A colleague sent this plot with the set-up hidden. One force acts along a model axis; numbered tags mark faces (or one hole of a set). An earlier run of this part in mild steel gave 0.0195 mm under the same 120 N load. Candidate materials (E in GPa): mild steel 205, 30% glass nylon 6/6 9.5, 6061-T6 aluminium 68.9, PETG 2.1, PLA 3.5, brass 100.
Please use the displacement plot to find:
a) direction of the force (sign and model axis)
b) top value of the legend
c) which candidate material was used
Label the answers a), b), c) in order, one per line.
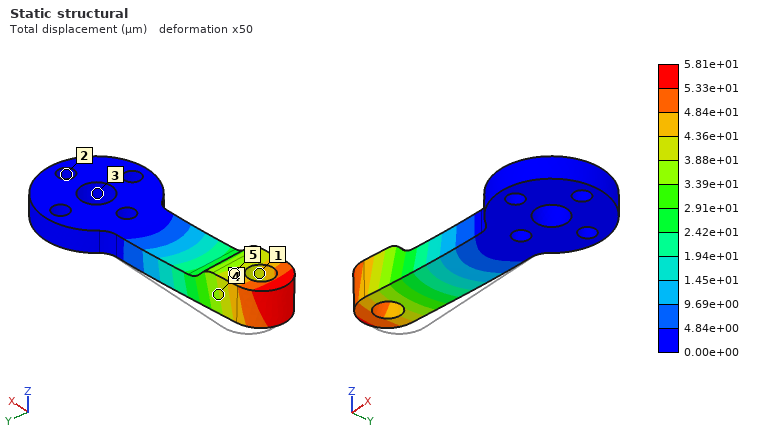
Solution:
a) -Y
b) 5.81e+01 µm
c) 6061-T6 aluminium
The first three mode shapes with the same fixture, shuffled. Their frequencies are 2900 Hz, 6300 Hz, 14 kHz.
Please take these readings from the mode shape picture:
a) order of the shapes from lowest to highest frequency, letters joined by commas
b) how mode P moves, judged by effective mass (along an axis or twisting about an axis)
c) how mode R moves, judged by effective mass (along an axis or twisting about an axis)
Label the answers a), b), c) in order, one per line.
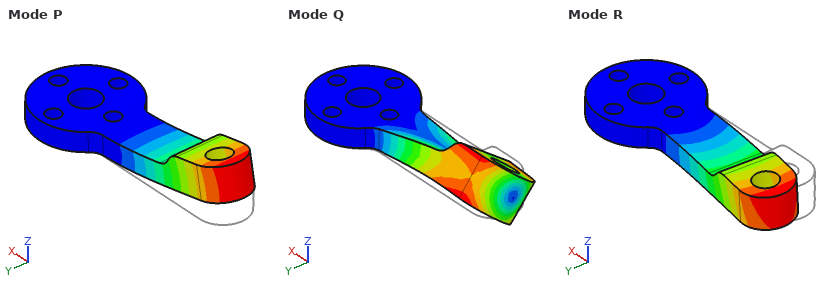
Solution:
a) P, R, Q
b) along Z
c) along Y
